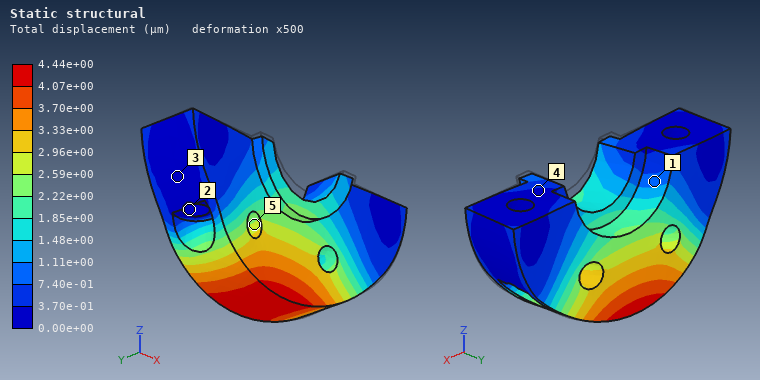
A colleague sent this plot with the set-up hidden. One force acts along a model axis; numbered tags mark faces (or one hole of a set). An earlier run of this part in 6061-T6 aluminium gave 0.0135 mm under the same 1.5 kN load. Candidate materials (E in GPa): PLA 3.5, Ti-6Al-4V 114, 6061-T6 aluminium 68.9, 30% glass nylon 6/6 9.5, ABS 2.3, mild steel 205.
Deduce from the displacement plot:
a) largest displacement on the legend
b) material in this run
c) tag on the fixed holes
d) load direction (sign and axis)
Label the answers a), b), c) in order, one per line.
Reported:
a) 4.44e+00 µm
b) mild steel
c) 2
d) +Y
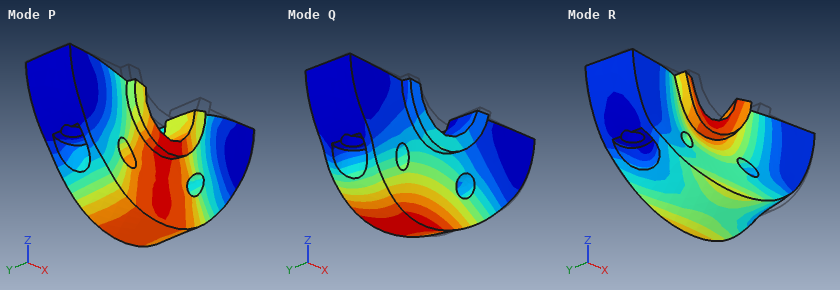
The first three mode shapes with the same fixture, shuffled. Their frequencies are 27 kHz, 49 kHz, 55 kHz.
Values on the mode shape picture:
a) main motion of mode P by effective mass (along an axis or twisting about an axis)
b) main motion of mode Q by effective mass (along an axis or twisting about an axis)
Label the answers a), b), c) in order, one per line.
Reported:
a) along Z
b) along Y
